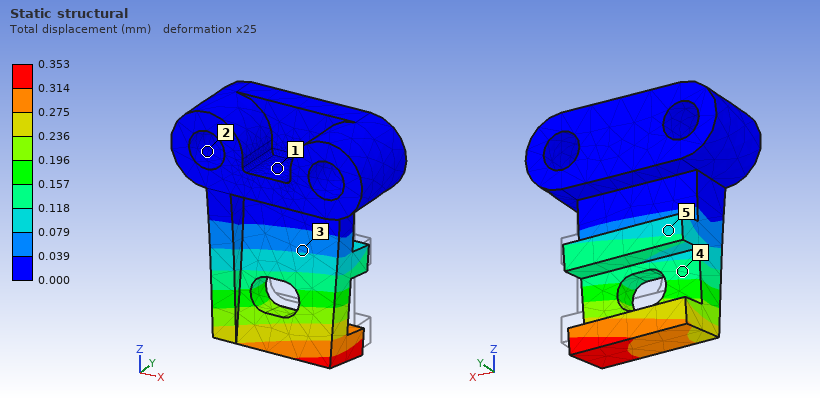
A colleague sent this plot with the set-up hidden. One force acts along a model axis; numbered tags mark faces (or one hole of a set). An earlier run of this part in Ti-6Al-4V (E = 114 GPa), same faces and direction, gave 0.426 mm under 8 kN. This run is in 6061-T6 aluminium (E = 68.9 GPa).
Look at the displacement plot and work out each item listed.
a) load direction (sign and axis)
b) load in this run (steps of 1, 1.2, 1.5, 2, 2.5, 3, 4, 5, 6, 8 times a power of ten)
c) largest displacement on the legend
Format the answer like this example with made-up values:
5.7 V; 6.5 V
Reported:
-Y; 4 kN; 0.353 mm
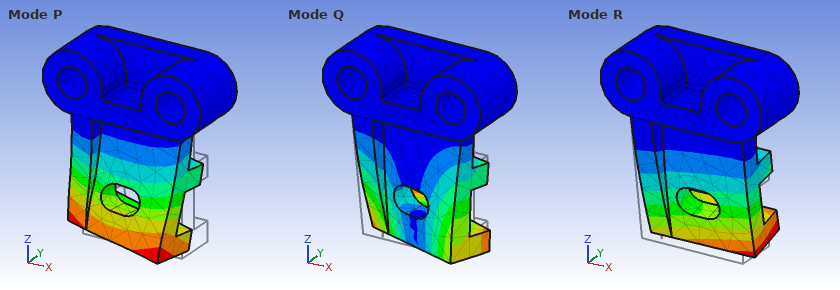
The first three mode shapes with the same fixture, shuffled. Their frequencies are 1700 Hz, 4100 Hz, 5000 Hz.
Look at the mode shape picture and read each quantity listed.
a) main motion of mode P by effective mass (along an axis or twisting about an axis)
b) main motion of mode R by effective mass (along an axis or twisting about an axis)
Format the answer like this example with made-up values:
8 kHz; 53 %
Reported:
along X; along Y
